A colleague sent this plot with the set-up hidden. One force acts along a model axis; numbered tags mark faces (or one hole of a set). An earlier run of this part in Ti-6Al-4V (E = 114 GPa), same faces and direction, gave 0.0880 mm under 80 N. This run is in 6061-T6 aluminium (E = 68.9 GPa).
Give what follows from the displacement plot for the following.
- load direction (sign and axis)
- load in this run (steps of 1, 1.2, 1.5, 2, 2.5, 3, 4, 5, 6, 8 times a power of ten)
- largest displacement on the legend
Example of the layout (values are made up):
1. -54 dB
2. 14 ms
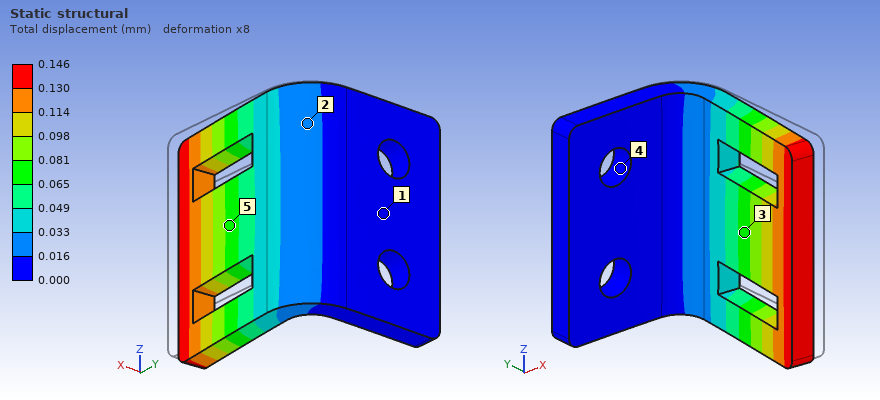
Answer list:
1. -X
2. 80 N
3. 0.146 mm
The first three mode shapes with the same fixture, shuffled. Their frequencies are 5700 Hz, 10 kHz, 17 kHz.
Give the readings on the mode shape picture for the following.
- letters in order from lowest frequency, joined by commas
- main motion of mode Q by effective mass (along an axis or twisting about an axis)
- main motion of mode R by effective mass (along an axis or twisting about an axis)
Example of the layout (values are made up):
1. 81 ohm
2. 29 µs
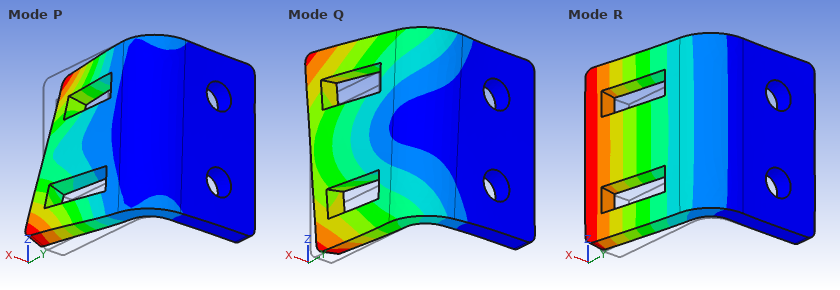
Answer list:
1. R, Q, P
2. along Z
3. along X
